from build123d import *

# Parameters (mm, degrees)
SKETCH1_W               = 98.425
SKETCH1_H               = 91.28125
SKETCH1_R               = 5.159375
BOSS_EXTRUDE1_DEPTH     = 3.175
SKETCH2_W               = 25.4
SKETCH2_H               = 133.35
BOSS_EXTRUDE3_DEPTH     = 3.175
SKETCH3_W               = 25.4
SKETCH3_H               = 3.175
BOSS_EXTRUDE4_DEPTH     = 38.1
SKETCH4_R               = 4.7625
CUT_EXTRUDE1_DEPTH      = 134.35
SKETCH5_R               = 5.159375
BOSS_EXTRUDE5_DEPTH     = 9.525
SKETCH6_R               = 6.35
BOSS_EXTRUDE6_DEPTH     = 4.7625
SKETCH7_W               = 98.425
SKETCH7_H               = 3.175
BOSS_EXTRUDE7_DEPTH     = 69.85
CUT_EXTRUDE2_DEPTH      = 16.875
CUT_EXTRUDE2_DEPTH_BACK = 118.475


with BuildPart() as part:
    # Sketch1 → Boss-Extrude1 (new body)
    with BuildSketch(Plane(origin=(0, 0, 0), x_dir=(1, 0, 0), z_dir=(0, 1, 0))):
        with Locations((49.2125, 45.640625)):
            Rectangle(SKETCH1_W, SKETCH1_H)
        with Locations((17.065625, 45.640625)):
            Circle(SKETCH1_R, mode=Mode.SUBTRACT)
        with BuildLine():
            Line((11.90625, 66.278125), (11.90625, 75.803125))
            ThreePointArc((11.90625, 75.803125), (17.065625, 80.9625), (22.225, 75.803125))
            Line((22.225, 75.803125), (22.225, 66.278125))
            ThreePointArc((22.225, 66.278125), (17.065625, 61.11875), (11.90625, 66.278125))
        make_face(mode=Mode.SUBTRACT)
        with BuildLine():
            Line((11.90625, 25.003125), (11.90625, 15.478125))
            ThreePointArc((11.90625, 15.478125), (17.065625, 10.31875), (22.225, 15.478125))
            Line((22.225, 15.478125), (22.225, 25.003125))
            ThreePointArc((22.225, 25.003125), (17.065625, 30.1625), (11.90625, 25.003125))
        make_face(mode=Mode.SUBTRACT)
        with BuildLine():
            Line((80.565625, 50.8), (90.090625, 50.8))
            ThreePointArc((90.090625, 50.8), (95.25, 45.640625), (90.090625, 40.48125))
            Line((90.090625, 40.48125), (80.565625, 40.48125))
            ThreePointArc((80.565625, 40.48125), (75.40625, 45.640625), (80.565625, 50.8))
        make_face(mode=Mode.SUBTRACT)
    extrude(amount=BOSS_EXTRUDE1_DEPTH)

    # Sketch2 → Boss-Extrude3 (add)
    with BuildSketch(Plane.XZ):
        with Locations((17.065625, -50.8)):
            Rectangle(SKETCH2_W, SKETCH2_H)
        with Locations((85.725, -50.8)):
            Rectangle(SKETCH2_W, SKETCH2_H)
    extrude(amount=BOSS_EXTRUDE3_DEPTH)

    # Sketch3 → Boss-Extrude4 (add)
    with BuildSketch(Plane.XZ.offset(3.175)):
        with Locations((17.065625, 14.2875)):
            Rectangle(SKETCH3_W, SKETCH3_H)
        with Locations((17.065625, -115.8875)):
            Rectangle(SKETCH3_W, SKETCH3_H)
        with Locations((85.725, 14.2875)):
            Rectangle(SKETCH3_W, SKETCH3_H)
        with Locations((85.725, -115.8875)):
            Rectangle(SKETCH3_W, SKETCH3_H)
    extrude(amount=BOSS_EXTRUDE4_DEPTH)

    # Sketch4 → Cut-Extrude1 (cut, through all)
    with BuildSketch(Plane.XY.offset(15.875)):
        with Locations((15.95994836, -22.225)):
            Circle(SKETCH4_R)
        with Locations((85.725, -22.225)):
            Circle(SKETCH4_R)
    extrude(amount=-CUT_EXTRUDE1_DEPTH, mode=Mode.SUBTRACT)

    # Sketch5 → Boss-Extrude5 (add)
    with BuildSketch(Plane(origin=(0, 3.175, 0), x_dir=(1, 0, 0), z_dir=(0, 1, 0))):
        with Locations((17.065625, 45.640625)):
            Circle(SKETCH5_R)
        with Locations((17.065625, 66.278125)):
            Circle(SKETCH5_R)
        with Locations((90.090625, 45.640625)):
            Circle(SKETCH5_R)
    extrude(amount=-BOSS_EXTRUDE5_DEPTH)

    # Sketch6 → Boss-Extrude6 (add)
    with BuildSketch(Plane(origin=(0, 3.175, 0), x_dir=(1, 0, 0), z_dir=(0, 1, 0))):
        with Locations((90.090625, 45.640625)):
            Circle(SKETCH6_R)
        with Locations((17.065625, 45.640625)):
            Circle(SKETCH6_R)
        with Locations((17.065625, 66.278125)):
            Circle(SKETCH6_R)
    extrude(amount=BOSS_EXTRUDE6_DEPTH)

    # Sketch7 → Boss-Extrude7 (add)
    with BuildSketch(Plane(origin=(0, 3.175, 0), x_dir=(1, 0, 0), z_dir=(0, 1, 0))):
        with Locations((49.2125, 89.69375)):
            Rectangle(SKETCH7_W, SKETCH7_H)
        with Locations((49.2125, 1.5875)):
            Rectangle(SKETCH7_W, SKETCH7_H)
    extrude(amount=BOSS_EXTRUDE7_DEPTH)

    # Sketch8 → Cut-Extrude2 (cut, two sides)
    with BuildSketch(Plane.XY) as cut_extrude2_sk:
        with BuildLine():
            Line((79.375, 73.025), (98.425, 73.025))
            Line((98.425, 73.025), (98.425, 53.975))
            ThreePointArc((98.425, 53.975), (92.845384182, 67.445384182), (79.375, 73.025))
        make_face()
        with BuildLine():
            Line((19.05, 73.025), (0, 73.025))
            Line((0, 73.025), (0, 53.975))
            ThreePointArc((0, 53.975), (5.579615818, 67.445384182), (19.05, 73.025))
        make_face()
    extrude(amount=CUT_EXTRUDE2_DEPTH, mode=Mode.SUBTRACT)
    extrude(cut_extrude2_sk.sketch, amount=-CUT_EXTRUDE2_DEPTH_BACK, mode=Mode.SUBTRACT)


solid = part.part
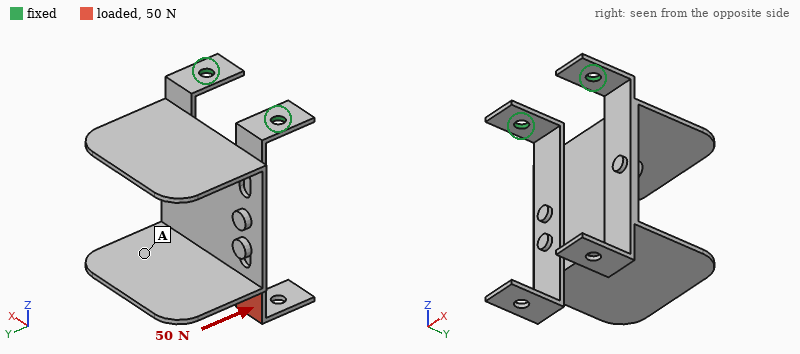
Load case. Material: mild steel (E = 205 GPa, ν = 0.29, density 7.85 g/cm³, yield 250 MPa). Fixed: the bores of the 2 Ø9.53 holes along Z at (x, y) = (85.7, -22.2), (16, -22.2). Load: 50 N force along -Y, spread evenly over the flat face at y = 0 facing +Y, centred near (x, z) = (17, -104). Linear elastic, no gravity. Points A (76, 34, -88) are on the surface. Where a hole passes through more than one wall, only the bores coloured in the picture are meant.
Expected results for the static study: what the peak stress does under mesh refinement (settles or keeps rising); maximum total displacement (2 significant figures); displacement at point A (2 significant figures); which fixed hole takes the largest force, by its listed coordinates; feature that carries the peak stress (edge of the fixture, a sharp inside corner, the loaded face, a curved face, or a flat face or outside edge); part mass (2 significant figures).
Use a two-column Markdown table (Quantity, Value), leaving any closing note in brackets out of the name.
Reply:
| Quantity | Value |
|---|---|
| what the peak stress does under mesh refinement | keeps rising |
| maximum total displacement | 0.93 mm |
| displacement at point A | 0.69 mm |
| which fixed hole takes the largest force, by its listed coordinates | (16, -22.2) |
| feature that carries the peak stress | edge of the fixture |
| part mass | 830 g |
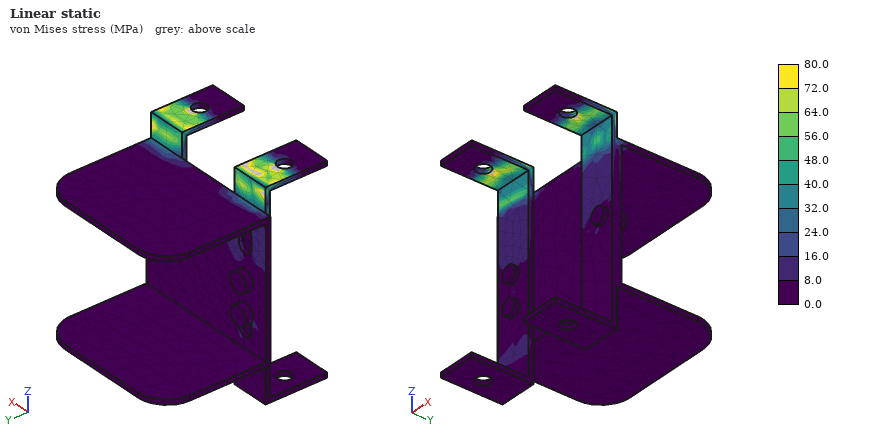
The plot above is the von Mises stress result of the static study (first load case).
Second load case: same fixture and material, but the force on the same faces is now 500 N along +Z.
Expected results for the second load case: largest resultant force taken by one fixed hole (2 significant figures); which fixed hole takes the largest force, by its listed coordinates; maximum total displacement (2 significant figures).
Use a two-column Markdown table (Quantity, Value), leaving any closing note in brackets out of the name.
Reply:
| Quantity | Value |
|---|---|
| largest resultant force taken by one fixed hole | 470 N |
| which fixed hole takes the largest force, by its listed coordinates | (16, -22.2) |
| maximum total displacement | 0.51 mm |
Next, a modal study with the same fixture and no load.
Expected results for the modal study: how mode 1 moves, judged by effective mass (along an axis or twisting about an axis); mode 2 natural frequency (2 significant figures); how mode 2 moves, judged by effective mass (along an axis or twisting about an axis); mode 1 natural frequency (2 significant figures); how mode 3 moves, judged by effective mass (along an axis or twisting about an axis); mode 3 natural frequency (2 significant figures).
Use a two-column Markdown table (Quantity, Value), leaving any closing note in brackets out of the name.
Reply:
| Quantity | Value |
|---|---|
| how mode 1 moves, judged by effective mass | along Y |
| mode 2 natural frequency | 340 Hz |
| how mode 2 moves, judged by effective mass | twisting about Z |
| mode 1 natural frequency | 67 Hz |
| how mode 3 moves, judged by effective mass | along X |
| mode 3 natural frequency | 420 Hz |
